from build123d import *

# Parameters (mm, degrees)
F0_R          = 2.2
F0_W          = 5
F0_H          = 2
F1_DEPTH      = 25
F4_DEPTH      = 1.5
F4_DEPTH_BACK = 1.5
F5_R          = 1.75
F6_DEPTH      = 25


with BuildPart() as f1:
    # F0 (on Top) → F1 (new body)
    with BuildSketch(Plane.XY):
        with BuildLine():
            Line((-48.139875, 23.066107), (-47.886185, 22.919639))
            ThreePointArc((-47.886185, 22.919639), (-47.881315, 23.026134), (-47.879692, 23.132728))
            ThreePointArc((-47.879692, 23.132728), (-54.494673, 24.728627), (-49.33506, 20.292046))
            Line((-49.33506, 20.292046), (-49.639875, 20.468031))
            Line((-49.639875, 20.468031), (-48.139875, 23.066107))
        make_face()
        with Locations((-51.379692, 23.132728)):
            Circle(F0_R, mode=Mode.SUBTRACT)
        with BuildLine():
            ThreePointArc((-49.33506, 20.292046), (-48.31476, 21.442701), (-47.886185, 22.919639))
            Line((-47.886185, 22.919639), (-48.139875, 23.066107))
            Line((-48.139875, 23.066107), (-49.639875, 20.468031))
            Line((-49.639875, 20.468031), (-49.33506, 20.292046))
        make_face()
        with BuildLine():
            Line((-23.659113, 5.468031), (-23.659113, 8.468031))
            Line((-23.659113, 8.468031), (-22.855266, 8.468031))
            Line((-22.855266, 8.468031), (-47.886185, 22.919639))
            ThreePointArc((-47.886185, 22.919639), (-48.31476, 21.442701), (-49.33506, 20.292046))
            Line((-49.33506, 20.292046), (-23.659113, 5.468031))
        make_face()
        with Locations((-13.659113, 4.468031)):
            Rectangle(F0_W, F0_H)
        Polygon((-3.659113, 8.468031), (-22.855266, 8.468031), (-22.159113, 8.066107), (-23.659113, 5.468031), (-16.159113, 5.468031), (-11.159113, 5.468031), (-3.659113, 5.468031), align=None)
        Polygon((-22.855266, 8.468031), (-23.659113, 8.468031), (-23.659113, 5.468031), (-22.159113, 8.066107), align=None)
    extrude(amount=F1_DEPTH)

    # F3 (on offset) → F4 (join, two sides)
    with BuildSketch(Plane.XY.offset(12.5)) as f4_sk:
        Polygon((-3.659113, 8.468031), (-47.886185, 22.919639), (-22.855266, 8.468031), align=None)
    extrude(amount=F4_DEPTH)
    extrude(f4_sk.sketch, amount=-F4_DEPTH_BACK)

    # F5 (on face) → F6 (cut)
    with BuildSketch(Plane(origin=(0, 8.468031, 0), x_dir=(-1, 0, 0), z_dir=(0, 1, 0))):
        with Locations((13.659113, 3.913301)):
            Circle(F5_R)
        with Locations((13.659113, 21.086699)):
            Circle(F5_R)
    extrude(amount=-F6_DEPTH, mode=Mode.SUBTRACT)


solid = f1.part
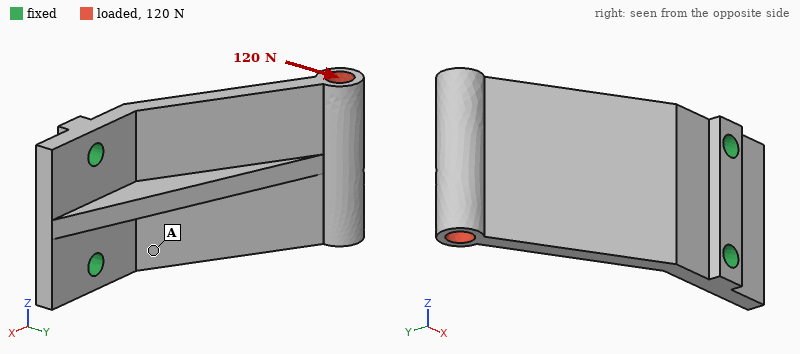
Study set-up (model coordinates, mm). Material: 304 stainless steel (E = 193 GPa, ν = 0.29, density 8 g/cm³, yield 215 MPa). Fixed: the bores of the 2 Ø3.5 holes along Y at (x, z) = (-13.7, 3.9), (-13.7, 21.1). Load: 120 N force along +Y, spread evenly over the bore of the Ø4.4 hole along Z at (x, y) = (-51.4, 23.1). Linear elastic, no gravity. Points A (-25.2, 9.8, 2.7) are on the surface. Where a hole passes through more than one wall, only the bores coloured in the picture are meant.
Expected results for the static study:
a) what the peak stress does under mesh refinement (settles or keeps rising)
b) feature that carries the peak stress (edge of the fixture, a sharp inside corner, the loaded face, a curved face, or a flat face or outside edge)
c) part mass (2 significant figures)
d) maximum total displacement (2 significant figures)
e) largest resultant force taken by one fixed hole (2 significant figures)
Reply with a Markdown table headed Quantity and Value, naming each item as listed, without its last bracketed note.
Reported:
| Quantity | Value |
|---|---|
| what the peak stress does under mesh refinement | keeps rising |
| feature that carries the peak stress | edge of the fixture |
| part mass | 38 g |
| maximum total displacement | 88 µm |
| largest resultant force taken by one fixed hole | 69 N |
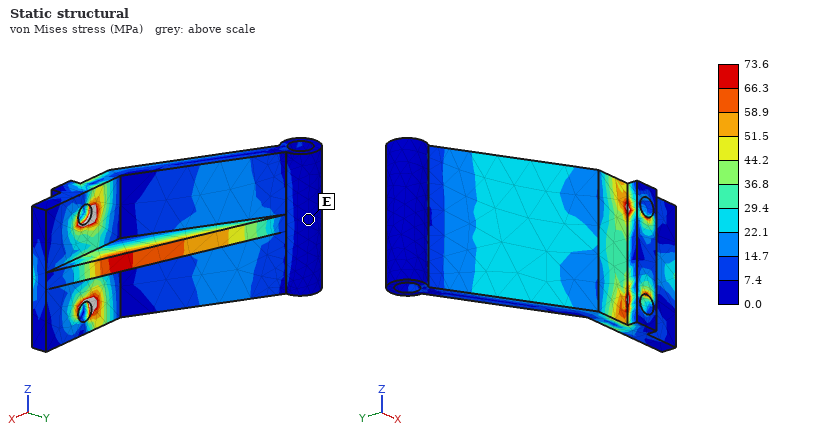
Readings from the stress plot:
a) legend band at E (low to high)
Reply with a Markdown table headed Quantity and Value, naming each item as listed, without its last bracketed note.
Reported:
| Quantity | Value |
|---|---|
| legend band at E | 0.0 to 7.4 MPa |
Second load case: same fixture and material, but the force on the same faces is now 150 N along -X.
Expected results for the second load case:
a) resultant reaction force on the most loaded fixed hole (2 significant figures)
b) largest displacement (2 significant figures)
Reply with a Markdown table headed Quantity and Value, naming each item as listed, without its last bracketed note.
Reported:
| Quantity | Value |
|---|---|
| resultant reaction force on the most loaded fixed hole | 75 N |
| largest displacement | 56 µm |
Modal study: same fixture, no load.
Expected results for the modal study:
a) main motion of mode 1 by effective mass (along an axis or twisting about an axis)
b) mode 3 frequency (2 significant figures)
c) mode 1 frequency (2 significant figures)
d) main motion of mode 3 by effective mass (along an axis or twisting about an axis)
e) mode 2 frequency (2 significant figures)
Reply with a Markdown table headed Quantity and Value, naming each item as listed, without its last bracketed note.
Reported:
| Quantity | Value |
|---|---|
| main motion of mode 1 by effective mass | along Y |
| mode 3 frequency | 6800 Hz |
| mode 1 frequency | 2000 Hz |
| main motion of mode 3 by effective mass | along Z |
| mode 2 frequency | 4700 Hz |
